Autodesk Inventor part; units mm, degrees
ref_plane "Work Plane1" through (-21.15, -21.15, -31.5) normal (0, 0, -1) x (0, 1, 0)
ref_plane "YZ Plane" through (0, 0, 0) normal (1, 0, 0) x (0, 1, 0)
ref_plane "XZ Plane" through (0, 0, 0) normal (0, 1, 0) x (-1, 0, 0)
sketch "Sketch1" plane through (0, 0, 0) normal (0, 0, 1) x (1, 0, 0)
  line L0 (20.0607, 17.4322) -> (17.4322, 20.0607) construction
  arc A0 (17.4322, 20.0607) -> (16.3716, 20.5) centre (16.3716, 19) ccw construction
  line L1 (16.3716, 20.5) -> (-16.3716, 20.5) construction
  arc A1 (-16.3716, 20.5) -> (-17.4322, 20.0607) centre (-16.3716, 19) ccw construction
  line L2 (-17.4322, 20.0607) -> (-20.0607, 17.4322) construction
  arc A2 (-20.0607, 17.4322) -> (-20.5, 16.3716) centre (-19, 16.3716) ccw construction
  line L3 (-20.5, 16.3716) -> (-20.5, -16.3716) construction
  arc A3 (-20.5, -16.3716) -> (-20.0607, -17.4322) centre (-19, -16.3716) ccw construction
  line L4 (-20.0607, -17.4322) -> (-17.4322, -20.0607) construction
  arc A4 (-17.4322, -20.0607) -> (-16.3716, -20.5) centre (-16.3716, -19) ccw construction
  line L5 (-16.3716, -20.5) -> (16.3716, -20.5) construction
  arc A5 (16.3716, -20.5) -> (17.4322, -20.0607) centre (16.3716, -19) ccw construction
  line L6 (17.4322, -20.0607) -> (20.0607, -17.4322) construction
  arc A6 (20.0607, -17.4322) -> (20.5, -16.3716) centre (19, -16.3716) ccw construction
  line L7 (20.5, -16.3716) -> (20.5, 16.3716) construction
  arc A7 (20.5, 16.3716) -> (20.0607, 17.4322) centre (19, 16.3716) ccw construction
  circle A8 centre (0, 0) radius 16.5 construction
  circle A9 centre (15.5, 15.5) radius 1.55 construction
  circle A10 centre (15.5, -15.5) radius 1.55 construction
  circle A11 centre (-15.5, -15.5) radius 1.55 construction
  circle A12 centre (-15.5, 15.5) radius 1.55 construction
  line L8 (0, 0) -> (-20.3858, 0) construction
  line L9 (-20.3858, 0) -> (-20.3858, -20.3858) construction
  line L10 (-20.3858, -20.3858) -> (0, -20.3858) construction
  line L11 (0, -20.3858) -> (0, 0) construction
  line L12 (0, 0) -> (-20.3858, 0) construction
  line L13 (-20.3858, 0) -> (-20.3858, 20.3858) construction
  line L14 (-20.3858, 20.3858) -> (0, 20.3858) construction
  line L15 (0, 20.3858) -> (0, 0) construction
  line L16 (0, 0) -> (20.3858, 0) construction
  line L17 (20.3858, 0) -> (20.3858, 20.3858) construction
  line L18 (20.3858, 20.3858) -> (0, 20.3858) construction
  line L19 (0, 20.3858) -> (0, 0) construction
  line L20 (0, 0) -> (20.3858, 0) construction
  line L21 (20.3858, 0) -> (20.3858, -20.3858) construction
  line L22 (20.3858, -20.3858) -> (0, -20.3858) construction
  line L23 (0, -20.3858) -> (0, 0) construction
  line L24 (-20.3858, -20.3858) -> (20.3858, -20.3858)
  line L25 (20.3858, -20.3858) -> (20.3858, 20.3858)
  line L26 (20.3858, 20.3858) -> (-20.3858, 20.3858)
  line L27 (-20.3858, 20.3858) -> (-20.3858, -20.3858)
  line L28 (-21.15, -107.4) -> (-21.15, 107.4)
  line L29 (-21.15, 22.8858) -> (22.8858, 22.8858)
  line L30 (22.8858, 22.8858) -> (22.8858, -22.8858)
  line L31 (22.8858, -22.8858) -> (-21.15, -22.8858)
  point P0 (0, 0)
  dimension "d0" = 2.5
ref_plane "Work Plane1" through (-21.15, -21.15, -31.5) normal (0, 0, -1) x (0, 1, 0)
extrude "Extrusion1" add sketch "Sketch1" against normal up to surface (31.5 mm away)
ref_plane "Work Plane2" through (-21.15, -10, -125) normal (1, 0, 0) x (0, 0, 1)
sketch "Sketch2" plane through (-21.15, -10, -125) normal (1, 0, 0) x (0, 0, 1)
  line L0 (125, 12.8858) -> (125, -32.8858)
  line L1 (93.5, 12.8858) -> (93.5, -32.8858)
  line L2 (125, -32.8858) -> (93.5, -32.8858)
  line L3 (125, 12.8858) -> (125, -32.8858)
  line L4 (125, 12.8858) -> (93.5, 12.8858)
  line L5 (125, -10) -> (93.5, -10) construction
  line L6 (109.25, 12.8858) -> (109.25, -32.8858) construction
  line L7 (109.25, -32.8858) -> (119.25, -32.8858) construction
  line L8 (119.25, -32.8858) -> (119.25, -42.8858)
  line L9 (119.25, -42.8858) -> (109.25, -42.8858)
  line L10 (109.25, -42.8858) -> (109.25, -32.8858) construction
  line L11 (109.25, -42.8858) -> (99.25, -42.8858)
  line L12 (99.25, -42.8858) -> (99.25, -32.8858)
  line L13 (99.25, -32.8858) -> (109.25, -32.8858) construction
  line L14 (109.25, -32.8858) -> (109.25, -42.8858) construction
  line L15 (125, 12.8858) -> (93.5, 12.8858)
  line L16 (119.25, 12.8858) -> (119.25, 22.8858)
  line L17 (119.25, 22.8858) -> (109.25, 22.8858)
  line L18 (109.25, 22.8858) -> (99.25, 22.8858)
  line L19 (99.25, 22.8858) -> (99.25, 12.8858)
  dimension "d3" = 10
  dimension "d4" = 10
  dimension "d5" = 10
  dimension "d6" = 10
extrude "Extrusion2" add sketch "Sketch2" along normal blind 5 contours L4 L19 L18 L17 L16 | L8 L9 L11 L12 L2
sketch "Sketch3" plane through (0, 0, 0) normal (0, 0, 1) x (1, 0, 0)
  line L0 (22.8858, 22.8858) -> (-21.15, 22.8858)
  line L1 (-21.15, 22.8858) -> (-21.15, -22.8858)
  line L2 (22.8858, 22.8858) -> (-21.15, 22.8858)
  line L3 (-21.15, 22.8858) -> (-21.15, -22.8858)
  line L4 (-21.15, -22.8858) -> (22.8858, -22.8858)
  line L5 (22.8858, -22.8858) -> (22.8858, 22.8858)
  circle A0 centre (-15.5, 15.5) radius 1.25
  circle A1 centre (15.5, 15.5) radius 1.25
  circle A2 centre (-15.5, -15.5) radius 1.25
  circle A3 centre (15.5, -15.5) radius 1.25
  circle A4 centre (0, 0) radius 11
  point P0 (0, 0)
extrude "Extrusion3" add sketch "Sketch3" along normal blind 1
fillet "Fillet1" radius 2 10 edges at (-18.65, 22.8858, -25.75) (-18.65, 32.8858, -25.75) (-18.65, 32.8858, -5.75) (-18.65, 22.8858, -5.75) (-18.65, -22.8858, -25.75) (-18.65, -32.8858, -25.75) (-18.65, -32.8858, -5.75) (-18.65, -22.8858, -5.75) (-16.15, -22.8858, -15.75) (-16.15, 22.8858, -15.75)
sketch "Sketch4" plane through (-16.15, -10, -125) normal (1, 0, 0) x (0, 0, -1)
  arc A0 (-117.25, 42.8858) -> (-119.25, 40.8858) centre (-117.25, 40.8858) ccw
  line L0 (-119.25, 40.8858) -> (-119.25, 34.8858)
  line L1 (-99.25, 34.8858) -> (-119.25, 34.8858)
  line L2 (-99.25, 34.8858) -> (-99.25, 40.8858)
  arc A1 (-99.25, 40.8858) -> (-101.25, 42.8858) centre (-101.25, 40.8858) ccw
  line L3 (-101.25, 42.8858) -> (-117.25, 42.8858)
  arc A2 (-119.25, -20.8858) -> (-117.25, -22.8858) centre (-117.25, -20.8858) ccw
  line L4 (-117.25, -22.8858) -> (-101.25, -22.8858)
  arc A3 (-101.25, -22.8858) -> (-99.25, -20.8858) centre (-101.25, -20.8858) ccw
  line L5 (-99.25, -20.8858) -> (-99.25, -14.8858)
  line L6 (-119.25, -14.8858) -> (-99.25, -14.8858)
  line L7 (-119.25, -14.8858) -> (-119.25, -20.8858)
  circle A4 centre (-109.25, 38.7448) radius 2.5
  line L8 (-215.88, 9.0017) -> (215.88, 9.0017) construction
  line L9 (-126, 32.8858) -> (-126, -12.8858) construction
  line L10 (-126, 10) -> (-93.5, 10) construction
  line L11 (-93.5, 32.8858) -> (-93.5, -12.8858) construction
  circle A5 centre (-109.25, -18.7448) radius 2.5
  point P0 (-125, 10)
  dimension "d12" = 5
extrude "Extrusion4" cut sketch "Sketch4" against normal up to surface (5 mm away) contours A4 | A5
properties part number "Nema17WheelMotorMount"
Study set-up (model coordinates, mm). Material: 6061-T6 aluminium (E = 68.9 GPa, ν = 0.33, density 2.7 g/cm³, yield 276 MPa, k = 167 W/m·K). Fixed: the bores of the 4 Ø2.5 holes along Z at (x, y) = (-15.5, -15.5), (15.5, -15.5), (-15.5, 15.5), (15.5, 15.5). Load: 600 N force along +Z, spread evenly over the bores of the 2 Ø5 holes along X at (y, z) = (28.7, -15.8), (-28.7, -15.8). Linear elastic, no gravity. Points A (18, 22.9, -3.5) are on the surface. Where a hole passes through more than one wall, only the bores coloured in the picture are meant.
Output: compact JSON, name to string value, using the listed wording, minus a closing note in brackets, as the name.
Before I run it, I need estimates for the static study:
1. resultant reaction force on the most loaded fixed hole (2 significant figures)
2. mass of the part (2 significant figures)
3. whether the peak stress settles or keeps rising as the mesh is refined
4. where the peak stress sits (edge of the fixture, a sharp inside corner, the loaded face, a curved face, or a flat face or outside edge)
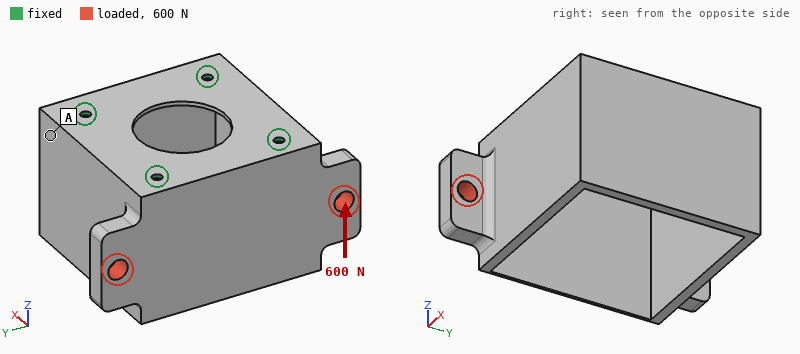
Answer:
{"resultant reaction force on the most loaded fixed hole": "340 N", "mass of the part": "39 g", "whether the peak stress settles or keeps rising as the mesh is refined": "keeps rising", "where the peak stress sits": "edge of the fixture"}
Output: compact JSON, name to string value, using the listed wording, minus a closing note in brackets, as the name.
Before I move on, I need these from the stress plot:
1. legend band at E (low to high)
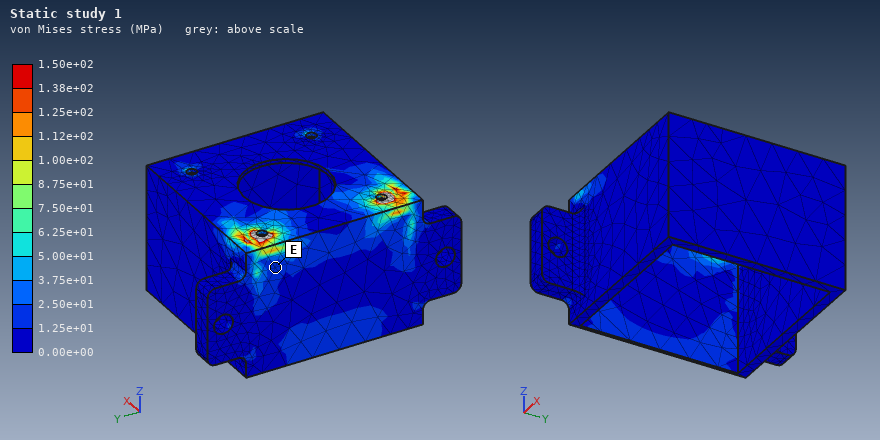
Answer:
{"legend band at E": "1.25e+01 to 2.50e+01 MPa"}
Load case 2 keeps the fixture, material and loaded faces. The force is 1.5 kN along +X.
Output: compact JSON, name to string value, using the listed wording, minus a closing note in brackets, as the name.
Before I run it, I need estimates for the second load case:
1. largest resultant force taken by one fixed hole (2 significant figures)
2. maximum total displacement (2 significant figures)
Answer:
{"largest resultant force taken by one fixed hole": "620 N", "maximum total displacement": "0.21 mm"}
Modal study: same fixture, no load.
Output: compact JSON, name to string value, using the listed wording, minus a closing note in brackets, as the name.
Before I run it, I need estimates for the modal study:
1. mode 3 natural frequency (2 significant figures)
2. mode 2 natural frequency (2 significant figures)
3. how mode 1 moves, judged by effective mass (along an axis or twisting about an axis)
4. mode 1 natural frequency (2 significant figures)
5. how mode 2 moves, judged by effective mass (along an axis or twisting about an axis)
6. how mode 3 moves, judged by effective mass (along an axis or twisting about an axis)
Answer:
{"mode 3 natural frequency": "2900 Hz", "mode 2 natural frequency": "2700 Hz", "how mode 1 moves, judged by effective mass": "along X", "mode 1 natural frequency": "2600 Hz", "how mode 2 moves, judged by effective mass": "along Y", "how mode 3 moves, judged by effective mass": "along Y"}
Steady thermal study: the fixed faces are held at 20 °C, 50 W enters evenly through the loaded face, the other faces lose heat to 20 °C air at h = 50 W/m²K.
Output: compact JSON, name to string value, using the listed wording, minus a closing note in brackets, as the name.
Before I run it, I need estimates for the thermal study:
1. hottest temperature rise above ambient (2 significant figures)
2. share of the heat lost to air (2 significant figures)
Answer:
{"hottest temperature rise above ambient": "56 K", "share of the heat lost to air": "33 %"}
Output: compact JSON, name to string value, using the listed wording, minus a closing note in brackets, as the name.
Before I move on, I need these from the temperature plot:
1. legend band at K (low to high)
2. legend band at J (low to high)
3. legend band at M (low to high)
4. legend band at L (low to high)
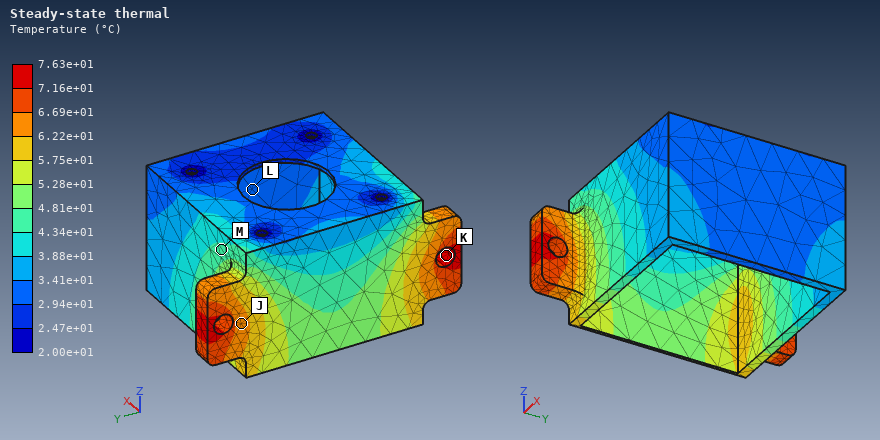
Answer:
{"legend band at K": "7.16e+01 to 7.63e+01 °C", "legend band at J": "6.22e+01 to 6.69e+01 °C", "legend band at M": "4.34e+01 to 4.81e+01 °C", "legend band at L": "2.94e+01 to 3.41e+01 °C"}
